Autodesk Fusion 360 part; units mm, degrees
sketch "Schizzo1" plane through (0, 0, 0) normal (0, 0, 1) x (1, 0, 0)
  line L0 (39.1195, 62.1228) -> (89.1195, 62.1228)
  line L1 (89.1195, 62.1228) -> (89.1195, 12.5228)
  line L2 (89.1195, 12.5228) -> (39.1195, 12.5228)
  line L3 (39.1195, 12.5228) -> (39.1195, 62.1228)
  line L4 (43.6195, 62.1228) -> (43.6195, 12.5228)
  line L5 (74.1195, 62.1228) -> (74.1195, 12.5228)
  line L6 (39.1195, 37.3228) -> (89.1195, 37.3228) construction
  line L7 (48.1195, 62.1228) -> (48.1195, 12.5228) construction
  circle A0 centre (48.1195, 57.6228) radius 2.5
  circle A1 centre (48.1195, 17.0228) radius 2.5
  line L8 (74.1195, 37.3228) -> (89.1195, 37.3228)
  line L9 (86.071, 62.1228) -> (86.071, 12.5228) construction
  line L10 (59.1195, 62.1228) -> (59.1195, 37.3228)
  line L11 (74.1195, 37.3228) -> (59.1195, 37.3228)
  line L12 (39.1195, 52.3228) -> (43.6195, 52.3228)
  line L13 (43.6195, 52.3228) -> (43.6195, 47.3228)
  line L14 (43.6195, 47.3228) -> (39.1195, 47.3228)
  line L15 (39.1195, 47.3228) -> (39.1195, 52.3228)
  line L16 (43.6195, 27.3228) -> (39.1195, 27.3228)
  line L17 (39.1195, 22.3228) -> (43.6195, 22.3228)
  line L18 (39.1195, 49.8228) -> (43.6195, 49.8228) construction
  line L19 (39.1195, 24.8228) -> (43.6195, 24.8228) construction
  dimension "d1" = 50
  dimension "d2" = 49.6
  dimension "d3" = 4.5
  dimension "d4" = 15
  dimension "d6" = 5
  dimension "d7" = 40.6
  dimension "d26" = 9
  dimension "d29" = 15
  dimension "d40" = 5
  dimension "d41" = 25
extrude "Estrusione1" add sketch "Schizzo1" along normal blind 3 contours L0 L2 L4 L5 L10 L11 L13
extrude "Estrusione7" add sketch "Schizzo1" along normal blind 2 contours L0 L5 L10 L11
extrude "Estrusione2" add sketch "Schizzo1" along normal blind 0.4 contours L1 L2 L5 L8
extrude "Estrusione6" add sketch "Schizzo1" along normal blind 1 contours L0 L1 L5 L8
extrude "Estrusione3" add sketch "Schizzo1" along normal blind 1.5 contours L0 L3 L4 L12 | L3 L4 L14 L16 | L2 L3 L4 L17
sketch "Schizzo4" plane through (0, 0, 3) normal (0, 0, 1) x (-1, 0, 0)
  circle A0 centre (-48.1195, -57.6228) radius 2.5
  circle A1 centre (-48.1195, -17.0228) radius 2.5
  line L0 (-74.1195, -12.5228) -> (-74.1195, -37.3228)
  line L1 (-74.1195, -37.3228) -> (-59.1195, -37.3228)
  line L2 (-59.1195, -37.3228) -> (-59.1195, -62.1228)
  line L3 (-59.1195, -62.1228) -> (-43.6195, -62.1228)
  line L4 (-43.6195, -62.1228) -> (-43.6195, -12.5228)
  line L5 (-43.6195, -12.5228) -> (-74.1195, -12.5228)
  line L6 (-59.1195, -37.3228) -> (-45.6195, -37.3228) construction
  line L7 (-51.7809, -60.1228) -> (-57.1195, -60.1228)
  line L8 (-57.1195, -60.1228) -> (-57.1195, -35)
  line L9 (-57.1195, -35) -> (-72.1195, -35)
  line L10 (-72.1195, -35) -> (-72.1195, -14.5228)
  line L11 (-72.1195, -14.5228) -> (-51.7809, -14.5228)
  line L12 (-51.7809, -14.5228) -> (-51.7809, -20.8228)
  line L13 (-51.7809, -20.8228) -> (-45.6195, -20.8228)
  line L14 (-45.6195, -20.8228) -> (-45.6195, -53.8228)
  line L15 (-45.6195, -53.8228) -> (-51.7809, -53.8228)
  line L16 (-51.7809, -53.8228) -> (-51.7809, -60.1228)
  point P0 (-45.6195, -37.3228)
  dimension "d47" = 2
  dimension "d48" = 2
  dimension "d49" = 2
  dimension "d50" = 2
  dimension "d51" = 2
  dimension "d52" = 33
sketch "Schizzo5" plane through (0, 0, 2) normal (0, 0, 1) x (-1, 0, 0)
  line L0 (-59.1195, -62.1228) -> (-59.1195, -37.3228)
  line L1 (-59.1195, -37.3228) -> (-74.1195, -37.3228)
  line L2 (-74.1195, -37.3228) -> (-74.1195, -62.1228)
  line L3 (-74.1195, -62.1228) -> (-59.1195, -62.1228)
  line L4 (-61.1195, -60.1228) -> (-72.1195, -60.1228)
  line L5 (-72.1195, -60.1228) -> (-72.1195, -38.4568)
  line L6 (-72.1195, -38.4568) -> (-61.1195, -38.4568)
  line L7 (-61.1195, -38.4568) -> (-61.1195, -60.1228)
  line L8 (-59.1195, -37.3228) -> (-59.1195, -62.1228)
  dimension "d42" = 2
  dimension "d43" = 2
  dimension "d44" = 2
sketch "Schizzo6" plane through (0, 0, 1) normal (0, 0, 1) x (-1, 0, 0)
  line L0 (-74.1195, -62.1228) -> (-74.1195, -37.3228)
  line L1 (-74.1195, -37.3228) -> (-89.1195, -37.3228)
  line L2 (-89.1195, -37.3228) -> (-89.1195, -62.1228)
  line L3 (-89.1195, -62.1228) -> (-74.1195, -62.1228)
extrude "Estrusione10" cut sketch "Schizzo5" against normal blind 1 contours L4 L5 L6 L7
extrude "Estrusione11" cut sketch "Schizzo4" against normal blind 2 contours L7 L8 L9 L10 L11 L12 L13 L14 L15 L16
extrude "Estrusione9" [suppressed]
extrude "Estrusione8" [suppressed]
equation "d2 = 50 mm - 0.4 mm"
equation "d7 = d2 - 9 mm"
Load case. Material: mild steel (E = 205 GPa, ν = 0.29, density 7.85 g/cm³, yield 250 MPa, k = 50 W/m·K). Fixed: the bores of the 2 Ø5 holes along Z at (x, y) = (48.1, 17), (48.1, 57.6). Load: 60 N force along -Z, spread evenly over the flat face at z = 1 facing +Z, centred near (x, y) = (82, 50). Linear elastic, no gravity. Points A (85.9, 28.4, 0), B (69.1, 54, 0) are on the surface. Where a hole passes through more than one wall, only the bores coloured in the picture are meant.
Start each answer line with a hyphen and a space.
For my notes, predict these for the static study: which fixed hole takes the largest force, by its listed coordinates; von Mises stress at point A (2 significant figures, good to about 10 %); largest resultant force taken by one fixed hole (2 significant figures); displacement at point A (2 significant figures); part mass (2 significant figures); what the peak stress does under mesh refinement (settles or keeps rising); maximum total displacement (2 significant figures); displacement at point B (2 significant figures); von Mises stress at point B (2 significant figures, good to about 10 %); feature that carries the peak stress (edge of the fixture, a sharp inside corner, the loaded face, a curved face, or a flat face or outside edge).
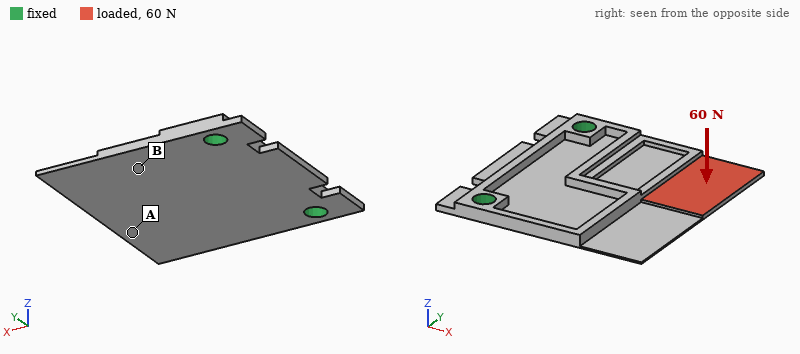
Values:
- (48.1, 57.6)
- 25 MPa
- 50 N
- 0.26 mm
- 24 g
- keeps rising
- 0.45 mm
- 0.12 mm
- 65 MPa
- a sharp inside corner
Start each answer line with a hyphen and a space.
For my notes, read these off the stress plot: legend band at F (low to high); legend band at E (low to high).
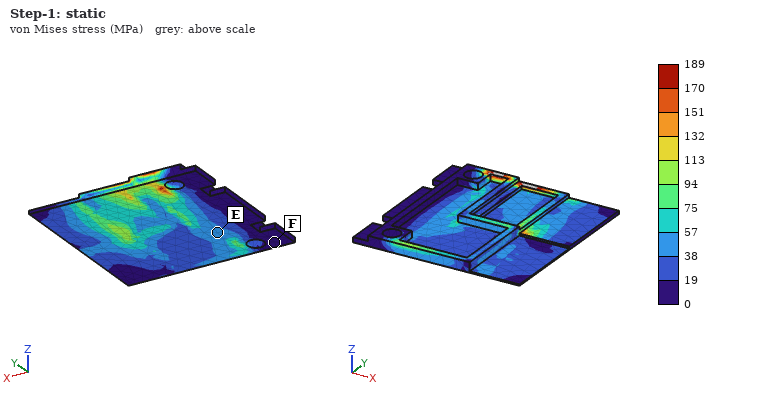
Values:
- 0 to 19 MPa
- 38 to 57 MPa
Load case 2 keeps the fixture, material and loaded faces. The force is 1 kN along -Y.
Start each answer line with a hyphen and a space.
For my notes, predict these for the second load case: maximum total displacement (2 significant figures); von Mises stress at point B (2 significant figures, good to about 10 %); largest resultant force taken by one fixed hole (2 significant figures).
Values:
- 0.17 mm
- 40 MPa
- 950 N
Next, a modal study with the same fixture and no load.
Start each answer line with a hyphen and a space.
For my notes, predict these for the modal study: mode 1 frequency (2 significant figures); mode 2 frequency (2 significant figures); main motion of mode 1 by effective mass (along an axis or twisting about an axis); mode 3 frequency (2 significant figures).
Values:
- 1000 Hz
- 1800 Hz
- along Z
- 2800 Hz
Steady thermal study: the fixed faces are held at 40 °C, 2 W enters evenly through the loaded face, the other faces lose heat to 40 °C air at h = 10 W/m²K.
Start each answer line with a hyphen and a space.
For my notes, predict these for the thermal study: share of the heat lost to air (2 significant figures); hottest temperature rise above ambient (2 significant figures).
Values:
- 24 %
- 31 K
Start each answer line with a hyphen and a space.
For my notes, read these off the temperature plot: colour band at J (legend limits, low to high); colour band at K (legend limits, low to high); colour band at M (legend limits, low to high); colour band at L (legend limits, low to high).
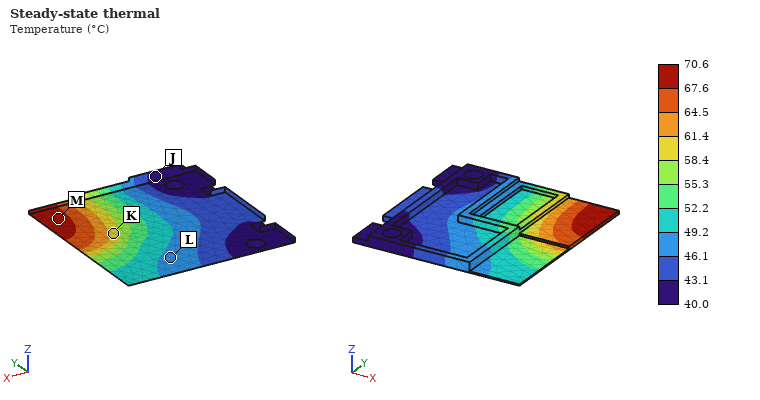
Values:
- 40.0 to 43.1 °C
- 58.4 to 61.4 °C
- 67.6 to 70.6 °C
- 46.1 to 49.2 °C
